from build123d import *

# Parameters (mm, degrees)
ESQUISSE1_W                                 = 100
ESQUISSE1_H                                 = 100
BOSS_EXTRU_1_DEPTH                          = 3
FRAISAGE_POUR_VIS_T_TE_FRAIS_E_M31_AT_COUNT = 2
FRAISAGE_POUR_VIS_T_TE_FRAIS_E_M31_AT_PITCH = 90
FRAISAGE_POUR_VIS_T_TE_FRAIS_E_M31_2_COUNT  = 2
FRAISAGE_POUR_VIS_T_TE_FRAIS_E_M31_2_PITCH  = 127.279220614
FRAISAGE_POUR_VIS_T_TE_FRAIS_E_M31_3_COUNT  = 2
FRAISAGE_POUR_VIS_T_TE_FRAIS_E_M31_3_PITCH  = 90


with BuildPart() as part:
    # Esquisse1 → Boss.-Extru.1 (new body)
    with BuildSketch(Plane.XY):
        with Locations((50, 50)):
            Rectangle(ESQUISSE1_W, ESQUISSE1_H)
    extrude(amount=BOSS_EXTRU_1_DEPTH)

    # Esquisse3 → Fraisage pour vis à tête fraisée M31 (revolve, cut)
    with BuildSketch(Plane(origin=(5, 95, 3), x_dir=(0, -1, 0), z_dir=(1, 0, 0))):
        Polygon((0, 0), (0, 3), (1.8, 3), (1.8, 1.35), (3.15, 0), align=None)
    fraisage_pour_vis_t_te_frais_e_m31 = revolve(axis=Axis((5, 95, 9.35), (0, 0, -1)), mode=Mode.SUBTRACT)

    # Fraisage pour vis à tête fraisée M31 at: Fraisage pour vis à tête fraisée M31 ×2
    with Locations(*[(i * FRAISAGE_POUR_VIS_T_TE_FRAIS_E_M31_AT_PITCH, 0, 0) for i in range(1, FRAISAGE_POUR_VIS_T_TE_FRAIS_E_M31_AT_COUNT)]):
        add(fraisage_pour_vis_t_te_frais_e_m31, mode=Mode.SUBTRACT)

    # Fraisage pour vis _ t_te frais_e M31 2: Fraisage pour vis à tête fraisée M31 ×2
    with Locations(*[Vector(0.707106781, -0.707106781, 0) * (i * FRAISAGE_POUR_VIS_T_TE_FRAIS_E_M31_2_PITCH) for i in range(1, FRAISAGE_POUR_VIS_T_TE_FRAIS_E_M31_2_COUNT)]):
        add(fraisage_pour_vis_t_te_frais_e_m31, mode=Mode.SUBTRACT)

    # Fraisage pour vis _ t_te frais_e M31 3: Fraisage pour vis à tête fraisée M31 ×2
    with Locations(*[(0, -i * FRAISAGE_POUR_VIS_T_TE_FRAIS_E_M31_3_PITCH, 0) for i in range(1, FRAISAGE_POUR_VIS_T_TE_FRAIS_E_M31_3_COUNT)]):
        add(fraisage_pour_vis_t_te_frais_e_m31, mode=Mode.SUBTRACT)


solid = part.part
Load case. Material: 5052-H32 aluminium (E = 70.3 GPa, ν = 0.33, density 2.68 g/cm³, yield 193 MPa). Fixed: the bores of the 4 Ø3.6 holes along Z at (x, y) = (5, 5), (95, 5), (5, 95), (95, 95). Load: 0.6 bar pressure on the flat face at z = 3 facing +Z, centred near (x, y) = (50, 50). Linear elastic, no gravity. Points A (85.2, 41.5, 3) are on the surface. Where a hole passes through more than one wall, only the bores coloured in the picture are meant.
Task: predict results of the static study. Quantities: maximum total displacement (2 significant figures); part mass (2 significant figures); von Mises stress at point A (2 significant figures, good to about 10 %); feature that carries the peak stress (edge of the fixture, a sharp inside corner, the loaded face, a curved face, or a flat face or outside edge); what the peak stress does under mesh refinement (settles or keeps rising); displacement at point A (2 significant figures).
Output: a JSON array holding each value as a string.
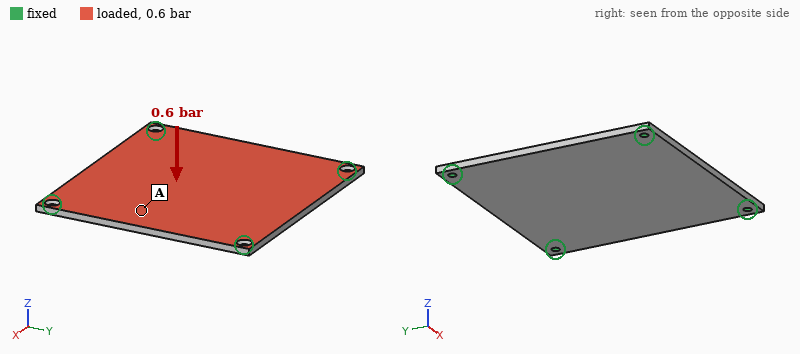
["0.23 mm", "80 g", "20 MPa", "edge of the fixture", "keeps rising", "0.15 mm"]
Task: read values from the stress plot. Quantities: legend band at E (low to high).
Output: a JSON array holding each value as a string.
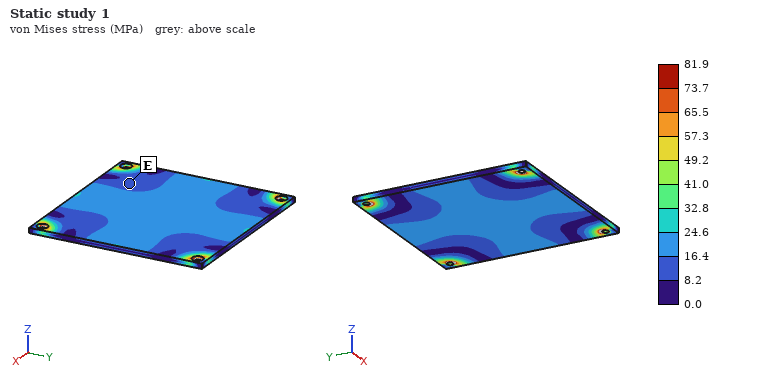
["8.2 to 16.4 MPa"]
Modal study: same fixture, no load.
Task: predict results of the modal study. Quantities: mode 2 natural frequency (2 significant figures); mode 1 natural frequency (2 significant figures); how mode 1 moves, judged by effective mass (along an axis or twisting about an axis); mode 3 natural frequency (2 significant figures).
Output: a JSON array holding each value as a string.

["2000 Hz", "1100 Hz", "along Z", "2000 Hz"]
